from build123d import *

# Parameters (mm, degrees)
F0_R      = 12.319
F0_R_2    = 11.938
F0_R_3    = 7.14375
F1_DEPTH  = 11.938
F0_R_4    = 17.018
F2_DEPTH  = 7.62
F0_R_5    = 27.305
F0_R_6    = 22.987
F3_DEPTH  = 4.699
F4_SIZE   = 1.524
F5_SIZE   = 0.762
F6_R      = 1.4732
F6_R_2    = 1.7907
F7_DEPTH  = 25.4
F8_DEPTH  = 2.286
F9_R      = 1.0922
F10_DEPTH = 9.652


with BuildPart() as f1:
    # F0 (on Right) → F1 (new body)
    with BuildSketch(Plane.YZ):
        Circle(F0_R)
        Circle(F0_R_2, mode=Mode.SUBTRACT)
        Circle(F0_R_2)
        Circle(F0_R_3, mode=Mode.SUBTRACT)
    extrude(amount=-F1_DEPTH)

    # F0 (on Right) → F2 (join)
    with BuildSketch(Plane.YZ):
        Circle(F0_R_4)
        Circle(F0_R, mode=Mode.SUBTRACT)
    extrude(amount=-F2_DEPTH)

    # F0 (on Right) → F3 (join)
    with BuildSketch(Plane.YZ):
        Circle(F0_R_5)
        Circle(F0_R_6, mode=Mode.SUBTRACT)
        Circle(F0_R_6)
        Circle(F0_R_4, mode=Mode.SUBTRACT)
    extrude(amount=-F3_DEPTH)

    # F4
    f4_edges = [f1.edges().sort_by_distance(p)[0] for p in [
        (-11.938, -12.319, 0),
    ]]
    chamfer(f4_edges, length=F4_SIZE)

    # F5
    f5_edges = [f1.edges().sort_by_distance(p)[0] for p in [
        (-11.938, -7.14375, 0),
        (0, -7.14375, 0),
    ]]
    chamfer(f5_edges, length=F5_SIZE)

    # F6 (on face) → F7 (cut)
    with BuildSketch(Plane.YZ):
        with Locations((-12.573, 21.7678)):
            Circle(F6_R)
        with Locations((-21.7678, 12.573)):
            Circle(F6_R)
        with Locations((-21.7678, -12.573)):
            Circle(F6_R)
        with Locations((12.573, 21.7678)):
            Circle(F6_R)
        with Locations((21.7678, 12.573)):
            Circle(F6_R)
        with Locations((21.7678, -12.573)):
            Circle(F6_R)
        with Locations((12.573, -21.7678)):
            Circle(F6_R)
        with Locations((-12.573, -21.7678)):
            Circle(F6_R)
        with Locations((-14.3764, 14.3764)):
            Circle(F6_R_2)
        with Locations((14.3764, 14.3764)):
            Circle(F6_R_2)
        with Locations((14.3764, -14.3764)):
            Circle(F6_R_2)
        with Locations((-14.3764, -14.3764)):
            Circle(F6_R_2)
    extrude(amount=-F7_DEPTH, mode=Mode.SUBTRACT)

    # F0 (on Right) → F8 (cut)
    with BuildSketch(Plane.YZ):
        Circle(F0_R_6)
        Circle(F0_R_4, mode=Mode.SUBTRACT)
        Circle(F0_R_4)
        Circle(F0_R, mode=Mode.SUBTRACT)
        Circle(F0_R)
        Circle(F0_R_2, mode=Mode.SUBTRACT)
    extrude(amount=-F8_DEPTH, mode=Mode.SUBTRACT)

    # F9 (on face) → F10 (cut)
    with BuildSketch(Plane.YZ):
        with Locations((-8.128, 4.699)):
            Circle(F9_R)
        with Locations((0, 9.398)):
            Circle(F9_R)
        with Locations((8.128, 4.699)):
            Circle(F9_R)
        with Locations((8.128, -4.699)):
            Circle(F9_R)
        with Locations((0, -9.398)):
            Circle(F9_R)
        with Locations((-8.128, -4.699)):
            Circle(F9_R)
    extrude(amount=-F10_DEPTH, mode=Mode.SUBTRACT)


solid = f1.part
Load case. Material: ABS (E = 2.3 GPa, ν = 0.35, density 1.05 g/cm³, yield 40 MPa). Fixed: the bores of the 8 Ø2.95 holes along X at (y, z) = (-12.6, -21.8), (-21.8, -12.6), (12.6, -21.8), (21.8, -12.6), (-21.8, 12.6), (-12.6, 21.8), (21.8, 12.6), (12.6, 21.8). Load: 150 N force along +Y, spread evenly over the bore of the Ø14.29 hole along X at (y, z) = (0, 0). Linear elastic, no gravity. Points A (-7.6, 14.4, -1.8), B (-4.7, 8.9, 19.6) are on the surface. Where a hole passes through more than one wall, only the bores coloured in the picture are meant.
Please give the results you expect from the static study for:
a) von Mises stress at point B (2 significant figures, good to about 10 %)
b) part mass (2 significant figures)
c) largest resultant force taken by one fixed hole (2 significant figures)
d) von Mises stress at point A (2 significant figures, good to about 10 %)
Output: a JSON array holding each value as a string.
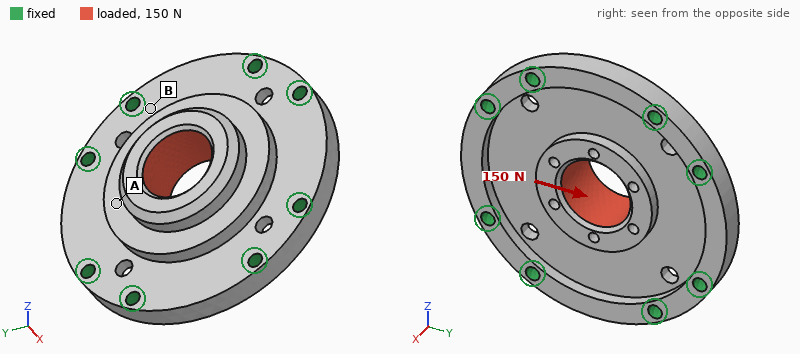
["0.78 MPa", "11 g", "25 N", "0.32 MPa"]
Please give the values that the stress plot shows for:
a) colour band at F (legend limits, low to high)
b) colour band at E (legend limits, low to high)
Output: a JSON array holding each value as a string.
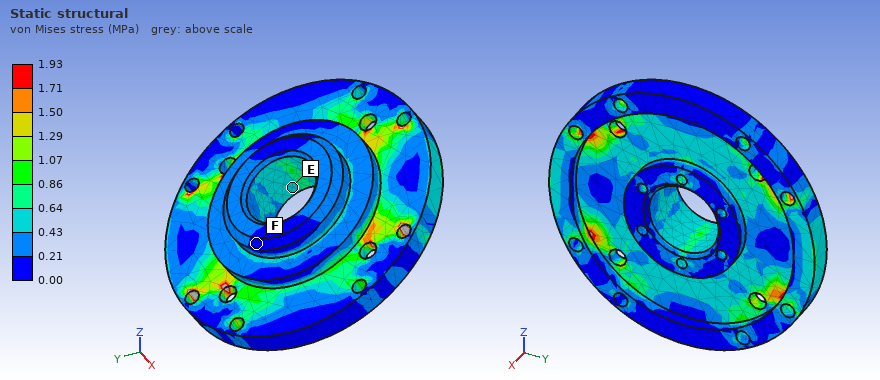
["0.00 to 0.21 MPa", "0.43 to 0.64 MPa"]
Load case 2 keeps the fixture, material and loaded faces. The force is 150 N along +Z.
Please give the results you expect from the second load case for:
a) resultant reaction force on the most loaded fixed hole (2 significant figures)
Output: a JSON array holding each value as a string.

["25 N"]
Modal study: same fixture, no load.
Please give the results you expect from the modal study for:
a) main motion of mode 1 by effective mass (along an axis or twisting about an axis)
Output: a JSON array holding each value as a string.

["along X"]
